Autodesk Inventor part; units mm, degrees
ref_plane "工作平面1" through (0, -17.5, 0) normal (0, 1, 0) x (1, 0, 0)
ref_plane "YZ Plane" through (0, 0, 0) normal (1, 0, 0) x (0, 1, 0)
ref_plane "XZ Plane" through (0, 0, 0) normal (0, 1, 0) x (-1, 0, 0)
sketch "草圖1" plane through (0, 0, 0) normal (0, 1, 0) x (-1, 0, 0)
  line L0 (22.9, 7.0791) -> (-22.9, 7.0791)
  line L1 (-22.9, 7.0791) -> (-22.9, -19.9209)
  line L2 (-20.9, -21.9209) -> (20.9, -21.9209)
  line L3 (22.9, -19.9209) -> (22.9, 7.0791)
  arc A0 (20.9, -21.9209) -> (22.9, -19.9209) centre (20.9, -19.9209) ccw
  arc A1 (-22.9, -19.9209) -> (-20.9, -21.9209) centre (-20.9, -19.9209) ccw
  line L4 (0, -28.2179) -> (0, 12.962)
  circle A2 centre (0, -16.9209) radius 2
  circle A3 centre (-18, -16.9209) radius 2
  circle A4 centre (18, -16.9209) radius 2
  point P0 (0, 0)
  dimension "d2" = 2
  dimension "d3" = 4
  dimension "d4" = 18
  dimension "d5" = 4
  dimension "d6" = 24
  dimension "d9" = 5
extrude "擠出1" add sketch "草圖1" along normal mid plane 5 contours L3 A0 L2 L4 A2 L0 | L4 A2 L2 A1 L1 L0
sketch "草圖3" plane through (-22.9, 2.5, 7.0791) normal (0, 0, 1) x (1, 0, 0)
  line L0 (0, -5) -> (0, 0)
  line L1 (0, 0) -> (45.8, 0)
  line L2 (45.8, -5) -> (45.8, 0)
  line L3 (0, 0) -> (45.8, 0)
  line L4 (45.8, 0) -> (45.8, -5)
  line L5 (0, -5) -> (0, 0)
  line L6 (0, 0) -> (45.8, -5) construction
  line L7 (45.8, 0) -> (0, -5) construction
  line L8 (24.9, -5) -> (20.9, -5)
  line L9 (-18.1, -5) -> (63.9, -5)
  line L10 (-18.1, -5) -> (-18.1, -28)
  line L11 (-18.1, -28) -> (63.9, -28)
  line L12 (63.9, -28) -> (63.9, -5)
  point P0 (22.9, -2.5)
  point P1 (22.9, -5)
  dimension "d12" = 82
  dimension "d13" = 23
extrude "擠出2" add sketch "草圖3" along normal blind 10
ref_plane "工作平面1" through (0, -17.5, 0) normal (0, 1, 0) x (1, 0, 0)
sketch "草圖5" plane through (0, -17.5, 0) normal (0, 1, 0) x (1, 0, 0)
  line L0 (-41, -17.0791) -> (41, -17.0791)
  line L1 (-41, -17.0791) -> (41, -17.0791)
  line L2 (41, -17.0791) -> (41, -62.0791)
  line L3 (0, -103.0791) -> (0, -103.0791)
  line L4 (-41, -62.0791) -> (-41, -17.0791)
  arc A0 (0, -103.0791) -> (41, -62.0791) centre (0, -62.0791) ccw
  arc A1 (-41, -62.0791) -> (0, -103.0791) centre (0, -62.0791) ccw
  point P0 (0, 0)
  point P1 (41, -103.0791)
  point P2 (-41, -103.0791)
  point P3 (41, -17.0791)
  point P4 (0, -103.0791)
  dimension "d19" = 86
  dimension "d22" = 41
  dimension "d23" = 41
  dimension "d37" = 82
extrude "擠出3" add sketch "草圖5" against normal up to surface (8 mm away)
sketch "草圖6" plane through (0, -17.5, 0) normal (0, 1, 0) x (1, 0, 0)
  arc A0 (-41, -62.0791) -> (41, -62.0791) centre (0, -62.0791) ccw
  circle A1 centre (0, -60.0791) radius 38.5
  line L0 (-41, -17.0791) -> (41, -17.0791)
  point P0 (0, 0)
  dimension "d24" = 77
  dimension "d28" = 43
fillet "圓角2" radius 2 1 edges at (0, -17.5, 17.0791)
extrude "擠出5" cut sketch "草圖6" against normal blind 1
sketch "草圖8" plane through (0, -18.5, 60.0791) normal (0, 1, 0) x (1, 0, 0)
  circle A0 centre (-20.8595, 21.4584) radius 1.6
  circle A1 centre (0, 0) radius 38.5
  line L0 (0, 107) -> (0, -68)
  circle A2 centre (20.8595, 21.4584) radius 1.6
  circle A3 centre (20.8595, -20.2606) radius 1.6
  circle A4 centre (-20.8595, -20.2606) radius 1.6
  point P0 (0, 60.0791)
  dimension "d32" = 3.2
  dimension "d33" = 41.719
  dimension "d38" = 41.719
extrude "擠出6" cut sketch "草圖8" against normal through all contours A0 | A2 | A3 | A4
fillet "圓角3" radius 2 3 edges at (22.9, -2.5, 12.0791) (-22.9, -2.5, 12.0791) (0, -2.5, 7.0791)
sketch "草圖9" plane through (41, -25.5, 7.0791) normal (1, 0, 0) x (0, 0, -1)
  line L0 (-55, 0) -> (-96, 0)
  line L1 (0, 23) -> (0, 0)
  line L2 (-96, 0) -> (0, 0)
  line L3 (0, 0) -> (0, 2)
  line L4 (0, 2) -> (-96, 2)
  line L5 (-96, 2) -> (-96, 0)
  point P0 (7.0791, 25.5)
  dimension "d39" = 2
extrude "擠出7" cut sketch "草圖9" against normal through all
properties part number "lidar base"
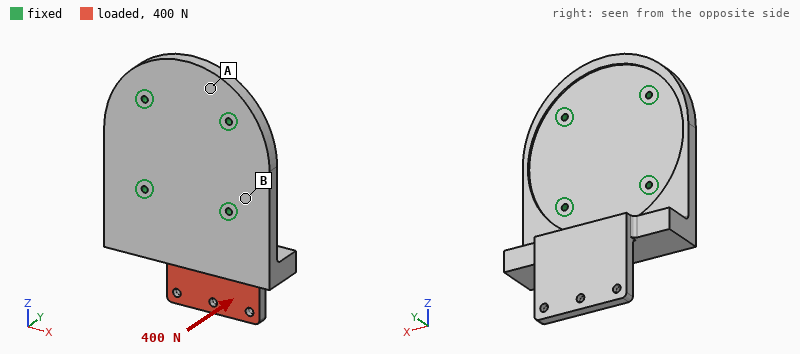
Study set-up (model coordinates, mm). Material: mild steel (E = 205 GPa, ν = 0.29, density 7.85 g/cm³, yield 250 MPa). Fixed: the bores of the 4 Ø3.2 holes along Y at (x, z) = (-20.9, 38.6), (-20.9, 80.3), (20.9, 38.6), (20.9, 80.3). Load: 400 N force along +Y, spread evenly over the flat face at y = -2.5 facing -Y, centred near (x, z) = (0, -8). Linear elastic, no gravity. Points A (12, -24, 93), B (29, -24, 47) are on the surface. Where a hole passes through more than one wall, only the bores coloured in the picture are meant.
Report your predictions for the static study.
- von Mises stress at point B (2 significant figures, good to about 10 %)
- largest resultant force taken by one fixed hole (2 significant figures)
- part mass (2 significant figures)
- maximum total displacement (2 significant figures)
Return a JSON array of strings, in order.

["13 MPa", "310 N", "470 g", "0.12 mm"]
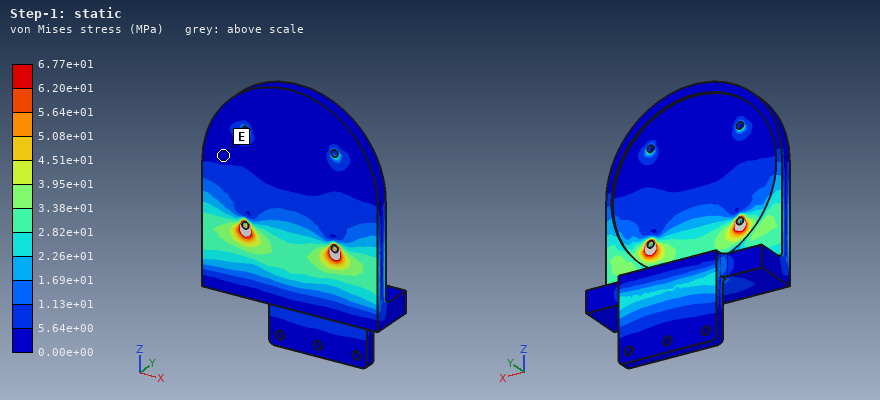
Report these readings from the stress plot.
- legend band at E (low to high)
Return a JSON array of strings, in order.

["0.00e+00 to 5.64e+00 MPa"]
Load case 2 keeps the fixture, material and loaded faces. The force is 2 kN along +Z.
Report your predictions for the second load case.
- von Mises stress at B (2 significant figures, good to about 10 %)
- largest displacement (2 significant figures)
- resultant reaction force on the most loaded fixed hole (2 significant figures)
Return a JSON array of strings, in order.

["25 MPa", "0.23 mm", "810 N"]
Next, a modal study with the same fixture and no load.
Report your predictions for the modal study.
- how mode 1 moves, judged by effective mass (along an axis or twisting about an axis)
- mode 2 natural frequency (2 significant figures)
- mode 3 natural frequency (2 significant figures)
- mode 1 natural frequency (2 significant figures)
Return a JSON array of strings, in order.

["along Y", "2900 Hz", "4900 Hz", "1100 Hz"]
